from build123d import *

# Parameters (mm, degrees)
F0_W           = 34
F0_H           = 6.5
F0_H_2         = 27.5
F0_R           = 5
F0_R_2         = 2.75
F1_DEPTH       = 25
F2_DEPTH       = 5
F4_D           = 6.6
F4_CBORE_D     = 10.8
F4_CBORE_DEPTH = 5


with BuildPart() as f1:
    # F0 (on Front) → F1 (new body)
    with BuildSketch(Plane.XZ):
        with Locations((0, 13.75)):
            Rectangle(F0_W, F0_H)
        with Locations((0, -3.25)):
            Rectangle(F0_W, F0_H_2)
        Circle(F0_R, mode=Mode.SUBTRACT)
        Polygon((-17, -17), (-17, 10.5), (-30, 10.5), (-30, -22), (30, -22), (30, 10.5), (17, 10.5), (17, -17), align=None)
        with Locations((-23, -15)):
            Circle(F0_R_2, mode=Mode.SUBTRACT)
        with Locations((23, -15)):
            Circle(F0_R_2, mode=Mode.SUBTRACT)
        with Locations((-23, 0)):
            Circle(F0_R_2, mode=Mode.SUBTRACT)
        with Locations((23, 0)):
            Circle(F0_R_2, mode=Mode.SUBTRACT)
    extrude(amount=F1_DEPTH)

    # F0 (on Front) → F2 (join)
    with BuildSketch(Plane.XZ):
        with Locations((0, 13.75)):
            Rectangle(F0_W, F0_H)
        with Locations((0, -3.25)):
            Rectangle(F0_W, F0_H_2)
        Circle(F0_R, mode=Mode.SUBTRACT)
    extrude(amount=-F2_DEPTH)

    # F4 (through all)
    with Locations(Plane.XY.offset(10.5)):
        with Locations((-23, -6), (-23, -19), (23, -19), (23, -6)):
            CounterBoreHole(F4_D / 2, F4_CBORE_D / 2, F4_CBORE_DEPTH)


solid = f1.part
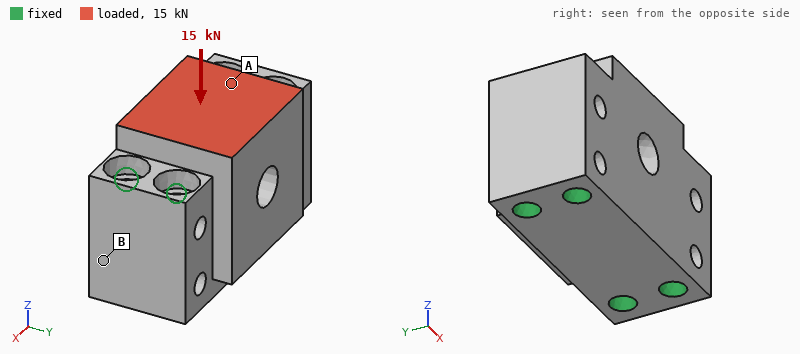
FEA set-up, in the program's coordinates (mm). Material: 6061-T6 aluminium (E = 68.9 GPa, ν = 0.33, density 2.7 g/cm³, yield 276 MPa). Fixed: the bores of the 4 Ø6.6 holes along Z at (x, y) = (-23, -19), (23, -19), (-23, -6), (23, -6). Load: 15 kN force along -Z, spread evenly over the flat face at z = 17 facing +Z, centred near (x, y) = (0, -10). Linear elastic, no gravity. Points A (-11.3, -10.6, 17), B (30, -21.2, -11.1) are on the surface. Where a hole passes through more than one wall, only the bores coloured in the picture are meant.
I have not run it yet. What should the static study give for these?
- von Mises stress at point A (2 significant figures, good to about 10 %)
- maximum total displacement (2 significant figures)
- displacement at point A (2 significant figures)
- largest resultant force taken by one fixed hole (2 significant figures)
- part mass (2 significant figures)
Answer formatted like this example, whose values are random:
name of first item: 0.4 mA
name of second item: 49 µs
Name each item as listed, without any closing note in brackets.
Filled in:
von Mises stress at point A: 16 MPa
maximum total displacement: 12 µm
displacement at point A: 7.8 µm
largest resultant force taken by one fixed hole: 4.7 kN
part mass: 140 g
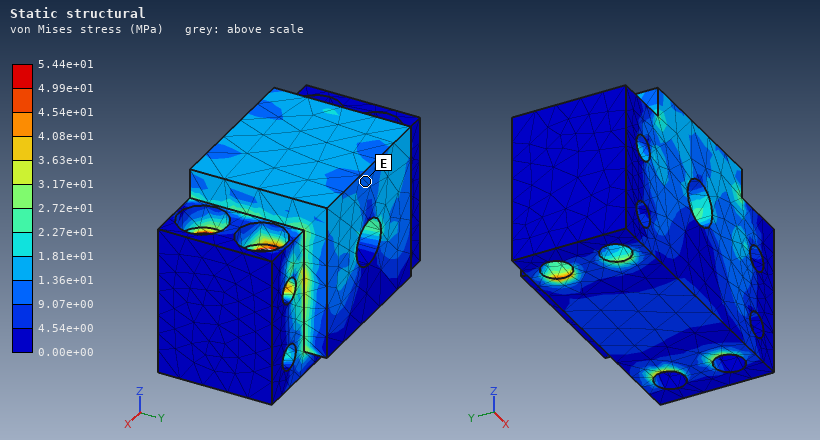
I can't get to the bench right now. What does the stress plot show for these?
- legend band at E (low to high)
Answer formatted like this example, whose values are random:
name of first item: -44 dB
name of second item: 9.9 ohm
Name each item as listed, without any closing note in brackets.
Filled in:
legend band at E: 9.07e+00 to 1.36e+01 MPa
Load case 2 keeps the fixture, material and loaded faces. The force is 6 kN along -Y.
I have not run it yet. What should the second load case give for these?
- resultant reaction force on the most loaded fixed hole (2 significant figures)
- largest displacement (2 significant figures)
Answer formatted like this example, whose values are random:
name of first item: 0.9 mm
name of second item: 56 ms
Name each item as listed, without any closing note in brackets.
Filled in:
resultant reaction force on the most loaded fixed hole: 3.1 kN
largest displacement: 20 µm
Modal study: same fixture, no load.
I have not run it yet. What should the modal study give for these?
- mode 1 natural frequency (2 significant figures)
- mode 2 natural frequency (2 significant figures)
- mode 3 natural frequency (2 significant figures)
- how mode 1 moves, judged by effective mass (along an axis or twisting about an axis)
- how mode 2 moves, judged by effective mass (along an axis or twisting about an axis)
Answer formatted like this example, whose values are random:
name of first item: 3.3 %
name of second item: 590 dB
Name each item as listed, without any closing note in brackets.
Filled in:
mode 1 natural frequency: 20 kHz
mode 2 natural frequency: 29 kHz
mode 3 natural frequency: 31 kHz
how mode 1 moves, judged by effective mass: along Y
how mode 2 moves, judged by effective mass: along Z
